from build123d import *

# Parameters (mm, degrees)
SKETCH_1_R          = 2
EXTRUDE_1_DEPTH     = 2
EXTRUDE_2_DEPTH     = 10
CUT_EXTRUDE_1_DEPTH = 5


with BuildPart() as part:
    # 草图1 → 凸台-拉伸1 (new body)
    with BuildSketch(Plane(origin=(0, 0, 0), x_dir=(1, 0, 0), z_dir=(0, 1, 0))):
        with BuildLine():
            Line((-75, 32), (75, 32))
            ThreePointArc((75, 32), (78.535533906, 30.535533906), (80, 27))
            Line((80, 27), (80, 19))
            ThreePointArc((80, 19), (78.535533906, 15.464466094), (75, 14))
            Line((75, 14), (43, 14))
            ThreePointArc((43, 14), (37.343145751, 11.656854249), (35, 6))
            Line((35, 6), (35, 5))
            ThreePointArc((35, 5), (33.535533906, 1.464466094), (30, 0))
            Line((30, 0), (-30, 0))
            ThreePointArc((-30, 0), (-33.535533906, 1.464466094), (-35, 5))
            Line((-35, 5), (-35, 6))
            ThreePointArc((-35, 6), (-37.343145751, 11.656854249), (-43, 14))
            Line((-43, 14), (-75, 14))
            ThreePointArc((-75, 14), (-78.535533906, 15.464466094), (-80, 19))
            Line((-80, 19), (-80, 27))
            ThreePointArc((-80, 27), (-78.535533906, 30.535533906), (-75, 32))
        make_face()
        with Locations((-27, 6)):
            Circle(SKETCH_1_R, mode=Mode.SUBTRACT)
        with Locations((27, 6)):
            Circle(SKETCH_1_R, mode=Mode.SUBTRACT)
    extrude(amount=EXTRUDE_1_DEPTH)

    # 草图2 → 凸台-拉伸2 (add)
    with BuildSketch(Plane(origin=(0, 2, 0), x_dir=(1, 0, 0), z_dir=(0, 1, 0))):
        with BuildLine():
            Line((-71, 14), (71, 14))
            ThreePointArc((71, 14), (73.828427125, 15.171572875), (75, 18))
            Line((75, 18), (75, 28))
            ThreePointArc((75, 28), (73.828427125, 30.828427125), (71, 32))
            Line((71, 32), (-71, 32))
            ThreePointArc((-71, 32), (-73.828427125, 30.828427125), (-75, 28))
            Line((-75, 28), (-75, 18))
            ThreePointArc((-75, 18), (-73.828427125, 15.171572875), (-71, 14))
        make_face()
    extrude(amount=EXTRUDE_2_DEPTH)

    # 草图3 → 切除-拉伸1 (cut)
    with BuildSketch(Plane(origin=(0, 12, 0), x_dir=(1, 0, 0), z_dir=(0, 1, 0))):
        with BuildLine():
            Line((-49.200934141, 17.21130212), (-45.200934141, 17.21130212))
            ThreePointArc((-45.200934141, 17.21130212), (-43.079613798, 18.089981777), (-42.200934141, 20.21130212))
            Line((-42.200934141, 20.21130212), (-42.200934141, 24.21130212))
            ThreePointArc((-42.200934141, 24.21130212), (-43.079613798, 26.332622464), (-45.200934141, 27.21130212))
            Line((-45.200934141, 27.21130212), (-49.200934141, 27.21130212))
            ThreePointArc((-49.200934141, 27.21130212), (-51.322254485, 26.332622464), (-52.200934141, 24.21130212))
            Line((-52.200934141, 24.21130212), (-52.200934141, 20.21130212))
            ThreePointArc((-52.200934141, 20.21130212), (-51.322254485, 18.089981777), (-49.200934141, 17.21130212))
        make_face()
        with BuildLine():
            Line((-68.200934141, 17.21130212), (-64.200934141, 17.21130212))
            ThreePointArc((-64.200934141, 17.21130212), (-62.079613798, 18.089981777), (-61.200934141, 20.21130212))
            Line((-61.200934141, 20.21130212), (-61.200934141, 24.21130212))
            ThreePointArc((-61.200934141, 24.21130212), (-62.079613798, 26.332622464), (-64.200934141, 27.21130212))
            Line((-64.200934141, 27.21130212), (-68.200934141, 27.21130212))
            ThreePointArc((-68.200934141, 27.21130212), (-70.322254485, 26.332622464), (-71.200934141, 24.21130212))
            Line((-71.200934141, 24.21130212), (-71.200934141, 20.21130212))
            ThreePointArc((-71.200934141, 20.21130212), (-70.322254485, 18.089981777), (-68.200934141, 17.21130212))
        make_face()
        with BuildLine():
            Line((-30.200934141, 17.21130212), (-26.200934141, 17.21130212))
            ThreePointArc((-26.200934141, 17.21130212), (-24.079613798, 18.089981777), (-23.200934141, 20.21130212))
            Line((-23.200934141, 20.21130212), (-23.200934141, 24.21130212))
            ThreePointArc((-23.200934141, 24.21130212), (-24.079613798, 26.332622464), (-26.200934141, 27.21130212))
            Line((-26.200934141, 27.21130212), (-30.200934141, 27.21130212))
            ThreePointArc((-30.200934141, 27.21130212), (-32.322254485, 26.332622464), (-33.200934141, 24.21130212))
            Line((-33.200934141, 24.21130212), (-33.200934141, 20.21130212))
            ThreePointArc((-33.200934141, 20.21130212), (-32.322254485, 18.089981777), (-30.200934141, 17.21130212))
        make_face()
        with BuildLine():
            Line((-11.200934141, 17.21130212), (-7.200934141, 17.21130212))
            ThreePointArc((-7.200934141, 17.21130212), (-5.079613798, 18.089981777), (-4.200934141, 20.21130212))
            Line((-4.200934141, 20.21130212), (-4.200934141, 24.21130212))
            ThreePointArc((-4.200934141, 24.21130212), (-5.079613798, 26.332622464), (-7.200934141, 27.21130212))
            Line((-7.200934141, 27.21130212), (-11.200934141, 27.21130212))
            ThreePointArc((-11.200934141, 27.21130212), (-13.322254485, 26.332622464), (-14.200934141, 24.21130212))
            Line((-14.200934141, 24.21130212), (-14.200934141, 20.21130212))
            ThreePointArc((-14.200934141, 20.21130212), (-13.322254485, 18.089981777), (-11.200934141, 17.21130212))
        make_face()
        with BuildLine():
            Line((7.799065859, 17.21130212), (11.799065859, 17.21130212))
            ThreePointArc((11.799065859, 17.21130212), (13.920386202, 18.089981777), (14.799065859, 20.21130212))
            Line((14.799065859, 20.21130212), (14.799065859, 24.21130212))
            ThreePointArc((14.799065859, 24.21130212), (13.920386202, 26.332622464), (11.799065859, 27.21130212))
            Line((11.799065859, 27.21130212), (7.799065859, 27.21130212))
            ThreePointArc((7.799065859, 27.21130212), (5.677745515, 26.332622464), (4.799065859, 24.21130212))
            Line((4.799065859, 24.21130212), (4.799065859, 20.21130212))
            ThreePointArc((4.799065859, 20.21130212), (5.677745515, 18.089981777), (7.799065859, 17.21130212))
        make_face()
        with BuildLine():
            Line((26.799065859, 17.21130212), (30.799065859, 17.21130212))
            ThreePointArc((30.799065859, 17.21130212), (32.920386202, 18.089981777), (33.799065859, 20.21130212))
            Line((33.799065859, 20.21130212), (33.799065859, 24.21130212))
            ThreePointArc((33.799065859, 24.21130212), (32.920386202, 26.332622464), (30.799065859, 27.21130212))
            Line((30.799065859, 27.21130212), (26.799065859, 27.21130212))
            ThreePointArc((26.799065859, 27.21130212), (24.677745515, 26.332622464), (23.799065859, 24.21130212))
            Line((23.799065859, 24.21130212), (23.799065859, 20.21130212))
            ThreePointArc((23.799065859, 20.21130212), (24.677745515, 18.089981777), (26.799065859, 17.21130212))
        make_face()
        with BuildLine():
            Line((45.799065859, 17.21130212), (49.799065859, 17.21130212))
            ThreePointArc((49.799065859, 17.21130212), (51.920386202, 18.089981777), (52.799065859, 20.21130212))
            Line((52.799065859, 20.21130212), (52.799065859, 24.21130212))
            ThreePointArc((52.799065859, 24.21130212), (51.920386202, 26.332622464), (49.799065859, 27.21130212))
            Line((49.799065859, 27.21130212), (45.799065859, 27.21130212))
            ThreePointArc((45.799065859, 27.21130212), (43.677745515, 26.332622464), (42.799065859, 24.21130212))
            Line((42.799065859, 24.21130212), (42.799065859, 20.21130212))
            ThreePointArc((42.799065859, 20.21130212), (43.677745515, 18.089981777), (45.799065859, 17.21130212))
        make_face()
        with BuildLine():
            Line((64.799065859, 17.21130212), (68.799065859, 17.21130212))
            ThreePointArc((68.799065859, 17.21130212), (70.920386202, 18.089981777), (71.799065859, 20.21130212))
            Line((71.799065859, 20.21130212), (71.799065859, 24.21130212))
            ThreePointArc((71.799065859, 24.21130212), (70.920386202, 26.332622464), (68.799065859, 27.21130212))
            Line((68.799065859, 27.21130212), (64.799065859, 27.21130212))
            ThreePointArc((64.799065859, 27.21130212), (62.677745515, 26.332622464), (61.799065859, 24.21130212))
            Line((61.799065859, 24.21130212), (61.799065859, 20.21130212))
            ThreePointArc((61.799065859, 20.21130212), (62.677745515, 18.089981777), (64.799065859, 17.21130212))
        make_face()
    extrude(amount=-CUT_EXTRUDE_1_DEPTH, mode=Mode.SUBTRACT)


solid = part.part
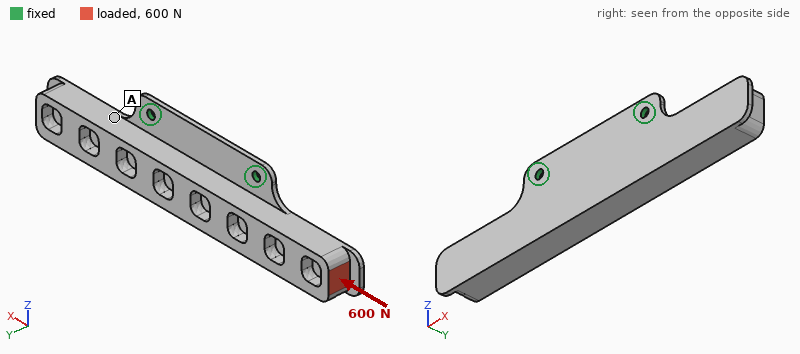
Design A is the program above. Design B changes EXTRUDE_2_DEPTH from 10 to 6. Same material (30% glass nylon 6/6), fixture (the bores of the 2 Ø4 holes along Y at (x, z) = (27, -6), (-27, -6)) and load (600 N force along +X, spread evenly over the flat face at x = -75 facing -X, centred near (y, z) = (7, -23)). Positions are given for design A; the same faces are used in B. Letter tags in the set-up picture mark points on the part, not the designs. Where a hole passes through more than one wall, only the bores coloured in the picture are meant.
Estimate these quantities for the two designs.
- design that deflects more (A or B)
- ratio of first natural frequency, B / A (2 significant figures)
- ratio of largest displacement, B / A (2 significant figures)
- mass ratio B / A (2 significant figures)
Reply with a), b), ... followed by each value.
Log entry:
a) B
b) 1.2
c) 1.2
d) 0.75
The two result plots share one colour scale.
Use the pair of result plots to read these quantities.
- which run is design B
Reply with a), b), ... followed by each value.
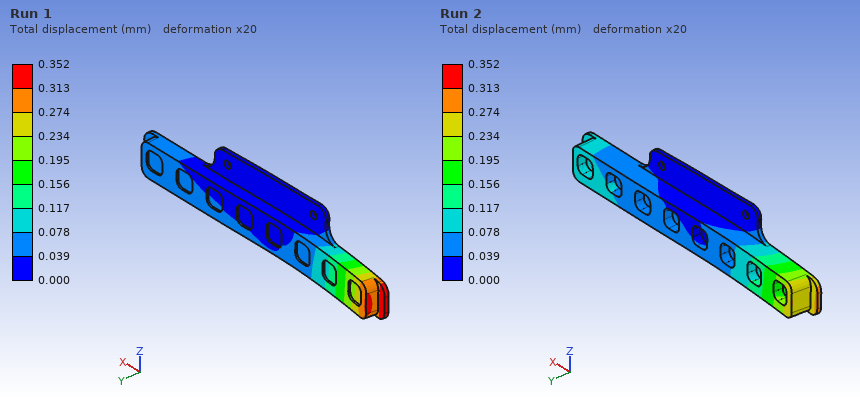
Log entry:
a) Run 1
